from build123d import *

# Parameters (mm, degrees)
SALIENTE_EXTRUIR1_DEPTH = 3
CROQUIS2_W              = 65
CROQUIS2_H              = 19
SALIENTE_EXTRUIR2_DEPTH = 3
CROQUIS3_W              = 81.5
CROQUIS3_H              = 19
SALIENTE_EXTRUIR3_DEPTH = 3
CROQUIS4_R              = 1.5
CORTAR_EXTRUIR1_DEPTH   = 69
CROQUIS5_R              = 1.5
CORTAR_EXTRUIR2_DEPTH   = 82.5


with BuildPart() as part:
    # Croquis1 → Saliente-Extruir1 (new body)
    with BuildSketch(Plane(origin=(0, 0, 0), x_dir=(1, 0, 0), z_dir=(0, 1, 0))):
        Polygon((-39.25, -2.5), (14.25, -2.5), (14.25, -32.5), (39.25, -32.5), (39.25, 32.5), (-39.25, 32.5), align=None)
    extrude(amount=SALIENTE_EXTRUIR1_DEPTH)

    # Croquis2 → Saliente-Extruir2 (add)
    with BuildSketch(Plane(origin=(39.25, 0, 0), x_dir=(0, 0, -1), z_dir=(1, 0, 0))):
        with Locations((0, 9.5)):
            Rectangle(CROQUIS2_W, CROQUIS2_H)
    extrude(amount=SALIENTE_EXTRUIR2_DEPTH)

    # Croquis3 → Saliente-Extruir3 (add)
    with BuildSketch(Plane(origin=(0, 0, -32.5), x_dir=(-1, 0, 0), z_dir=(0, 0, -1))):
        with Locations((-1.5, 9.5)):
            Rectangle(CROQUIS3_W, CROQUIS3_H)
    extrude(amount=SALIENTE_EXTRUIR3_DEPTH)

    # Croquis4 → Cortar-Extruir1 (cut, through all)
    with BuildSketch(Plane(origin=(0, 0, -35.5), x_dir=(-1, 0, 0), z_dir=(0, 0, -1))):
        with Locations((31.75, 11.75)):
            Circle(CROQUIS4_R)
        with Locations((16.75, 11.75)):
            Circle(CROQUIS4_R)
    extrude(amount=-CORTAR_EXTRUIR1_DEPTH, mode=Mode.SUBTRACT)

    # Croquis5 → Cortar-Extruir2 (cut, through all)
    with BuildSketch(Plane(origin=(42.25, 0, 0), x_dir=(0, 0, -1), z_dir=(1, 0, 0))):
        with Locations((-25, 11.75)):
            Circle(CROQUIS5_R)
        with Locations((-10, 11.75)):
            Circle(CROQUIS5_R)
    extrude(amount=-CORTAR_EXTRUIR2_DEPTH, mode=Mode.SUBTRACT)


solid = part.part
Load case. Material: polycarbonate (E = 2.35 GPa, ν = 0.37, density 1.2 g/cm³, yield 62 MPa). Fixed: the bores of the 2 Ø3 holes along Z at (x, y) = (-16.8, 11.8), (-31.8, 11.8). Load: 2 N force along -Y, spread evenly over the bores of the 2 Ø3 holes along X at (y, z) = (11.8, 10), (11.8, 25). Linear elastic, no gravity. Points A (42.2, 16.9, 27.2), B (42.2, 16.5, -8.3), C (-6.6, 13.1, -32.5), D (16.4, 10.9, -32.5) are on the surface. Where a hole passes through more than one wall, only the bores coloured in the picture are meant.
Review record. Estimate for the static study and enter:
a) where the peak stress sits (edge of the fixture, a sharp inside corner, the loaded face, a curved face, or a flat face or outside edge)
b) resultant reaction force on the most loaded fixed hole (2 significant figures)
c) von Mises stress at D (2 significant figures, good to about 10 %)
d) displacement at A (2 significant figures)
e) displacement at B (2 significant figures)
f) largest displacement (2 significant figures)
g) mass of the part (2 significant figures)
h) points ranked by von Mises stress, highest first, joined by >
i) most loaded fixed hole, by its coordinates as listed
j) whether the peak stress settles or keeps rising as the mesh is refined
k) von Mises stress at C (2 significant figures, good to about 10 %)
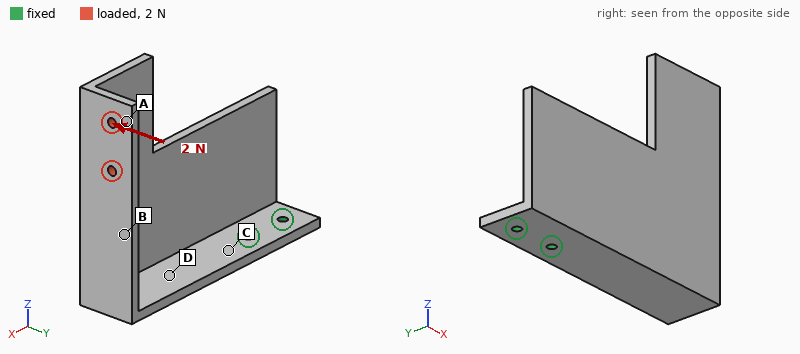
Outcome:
edge of the fixture
8.4 N
1.2 MPa
1.0 mm
0.46 mm
1.1 mm
23 g
C > D > B > A
(-16.8, 11.8)
keeps rising
1.7 MPa
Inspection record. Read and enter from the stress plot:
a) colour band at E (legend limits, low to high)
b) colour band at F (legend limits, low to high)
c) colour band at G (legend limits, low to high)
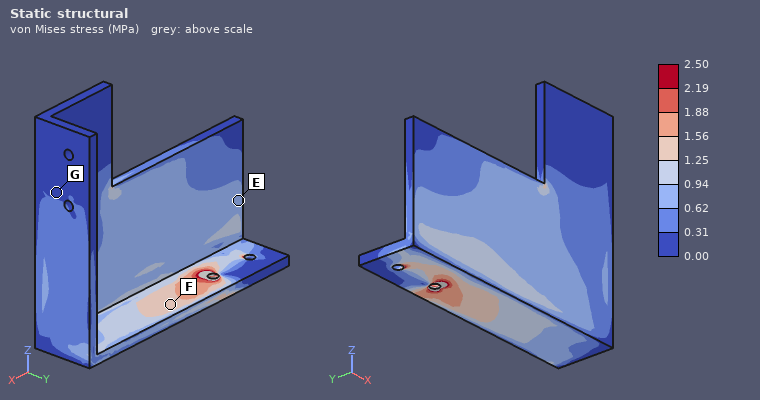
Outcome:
0.62 to 0.94 MPa
1.25 to 1.56 MPa
0.00 to 0.31 MPa
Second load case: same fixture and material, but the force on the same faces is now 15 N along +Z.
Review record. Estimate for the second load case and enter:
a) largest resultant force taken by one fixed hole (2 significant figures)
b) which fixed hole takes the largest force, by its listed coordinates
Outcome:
55 N
(-16.8, 11.8)
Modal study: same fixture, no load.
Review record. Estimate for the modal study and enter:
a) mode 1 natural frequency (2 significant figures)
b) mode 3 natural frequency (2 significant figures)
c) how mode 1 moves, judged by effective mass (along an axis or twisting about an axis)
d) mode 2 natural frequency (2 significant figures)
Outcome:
100 Hz
440 Hz
along Y
190 Hz
